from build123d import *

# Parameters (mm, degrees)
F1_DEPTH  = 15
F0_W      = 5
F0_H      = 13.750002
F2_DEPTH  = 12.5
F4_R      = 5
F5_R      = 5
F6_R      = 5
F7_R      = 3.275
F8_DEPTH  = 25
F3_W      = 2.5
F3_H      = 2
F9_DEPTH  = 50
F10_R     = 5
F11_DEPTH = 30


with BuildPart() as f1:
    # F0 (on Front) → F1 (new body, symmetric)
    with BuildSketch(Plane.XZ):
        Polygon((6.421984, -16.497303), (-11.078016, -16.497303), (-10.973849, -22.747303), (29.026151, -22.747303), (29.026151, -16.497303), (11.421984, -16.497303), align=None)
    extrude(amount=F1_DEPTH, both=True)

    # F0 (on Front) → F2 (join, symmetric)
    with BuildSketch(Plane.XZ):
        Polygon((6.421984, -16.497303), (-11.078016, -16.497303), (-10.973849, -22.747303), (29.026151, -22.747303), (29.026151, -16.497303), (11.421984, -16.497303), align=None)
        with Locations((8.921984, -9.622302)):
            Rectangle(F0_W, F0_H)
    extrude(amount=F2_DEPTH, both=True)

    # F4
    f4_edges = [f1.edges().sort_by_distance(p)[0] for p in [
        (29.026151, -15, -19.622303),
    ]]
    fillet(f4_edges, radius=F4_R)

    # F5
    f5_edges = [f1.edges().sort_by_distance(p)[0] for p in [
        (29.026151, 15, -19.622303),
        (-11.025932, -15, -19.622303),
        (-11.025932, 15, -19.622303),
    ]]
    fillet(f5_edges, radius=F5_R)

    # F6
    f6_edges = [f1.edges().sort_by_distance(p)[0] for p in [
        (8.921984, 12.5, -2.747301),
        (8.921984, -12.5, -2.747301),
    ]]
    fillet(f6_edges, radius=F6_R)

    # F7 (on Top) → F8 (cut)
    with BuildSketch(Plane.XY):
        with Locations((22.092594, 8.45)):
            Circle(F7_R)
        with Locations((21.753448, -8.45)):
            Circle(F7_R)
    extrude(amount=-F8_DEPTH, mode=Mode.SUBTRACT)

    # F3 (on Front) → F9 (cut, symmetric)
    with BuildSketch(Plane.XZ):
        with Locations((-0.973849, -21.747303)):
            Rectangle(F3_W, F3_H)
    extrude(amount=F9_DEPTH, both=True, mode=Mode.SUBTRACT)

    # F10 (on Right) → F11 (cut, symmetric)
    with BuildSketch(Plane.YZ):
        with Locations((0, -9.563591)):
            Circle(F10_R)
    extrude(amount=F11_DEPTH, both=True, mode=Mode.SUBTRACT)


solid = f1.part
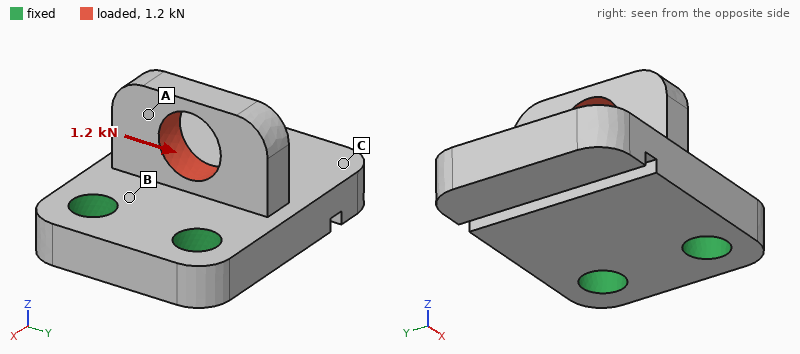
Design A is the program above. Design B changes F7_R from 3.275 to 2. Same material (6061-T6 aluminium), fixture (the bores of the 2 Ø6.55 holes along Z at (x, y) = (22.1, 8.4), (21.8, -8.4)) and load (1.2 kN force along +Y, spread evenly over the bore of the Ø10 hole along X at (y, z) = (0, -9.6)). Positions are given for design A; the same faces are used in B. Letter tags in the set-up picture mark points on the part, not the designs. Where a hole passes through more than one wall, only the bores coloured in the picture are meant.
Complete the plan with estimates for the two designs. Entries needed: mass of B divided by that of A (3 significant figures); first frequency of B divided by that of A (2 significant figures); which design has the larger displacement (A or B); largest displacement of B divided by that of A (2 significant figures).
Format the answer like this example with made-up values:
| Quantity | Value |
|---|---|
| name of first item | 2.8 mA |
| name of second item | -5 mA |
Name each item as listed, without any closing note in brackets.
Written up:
| Quantity | Value |
|---|---|
| mass of B divided by that of A | 1.03 |
| first frequency of B divided by that of A | 0.89 |
| which design has the larger displacement | B |
| largest displacement of B divided by that of A | 1.2 |
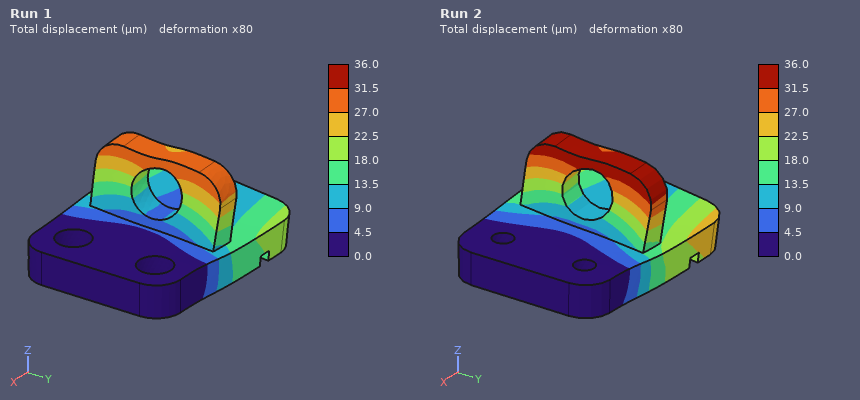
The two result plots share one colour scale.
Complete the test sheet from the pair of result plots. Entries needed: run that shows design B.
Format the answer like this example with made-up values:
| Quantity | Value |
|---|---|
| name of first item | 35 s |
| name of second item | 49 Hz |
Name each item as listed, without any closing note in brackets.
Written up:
| Quantity | Value |
|---|---|
| run that shows design B | Run 2 |
